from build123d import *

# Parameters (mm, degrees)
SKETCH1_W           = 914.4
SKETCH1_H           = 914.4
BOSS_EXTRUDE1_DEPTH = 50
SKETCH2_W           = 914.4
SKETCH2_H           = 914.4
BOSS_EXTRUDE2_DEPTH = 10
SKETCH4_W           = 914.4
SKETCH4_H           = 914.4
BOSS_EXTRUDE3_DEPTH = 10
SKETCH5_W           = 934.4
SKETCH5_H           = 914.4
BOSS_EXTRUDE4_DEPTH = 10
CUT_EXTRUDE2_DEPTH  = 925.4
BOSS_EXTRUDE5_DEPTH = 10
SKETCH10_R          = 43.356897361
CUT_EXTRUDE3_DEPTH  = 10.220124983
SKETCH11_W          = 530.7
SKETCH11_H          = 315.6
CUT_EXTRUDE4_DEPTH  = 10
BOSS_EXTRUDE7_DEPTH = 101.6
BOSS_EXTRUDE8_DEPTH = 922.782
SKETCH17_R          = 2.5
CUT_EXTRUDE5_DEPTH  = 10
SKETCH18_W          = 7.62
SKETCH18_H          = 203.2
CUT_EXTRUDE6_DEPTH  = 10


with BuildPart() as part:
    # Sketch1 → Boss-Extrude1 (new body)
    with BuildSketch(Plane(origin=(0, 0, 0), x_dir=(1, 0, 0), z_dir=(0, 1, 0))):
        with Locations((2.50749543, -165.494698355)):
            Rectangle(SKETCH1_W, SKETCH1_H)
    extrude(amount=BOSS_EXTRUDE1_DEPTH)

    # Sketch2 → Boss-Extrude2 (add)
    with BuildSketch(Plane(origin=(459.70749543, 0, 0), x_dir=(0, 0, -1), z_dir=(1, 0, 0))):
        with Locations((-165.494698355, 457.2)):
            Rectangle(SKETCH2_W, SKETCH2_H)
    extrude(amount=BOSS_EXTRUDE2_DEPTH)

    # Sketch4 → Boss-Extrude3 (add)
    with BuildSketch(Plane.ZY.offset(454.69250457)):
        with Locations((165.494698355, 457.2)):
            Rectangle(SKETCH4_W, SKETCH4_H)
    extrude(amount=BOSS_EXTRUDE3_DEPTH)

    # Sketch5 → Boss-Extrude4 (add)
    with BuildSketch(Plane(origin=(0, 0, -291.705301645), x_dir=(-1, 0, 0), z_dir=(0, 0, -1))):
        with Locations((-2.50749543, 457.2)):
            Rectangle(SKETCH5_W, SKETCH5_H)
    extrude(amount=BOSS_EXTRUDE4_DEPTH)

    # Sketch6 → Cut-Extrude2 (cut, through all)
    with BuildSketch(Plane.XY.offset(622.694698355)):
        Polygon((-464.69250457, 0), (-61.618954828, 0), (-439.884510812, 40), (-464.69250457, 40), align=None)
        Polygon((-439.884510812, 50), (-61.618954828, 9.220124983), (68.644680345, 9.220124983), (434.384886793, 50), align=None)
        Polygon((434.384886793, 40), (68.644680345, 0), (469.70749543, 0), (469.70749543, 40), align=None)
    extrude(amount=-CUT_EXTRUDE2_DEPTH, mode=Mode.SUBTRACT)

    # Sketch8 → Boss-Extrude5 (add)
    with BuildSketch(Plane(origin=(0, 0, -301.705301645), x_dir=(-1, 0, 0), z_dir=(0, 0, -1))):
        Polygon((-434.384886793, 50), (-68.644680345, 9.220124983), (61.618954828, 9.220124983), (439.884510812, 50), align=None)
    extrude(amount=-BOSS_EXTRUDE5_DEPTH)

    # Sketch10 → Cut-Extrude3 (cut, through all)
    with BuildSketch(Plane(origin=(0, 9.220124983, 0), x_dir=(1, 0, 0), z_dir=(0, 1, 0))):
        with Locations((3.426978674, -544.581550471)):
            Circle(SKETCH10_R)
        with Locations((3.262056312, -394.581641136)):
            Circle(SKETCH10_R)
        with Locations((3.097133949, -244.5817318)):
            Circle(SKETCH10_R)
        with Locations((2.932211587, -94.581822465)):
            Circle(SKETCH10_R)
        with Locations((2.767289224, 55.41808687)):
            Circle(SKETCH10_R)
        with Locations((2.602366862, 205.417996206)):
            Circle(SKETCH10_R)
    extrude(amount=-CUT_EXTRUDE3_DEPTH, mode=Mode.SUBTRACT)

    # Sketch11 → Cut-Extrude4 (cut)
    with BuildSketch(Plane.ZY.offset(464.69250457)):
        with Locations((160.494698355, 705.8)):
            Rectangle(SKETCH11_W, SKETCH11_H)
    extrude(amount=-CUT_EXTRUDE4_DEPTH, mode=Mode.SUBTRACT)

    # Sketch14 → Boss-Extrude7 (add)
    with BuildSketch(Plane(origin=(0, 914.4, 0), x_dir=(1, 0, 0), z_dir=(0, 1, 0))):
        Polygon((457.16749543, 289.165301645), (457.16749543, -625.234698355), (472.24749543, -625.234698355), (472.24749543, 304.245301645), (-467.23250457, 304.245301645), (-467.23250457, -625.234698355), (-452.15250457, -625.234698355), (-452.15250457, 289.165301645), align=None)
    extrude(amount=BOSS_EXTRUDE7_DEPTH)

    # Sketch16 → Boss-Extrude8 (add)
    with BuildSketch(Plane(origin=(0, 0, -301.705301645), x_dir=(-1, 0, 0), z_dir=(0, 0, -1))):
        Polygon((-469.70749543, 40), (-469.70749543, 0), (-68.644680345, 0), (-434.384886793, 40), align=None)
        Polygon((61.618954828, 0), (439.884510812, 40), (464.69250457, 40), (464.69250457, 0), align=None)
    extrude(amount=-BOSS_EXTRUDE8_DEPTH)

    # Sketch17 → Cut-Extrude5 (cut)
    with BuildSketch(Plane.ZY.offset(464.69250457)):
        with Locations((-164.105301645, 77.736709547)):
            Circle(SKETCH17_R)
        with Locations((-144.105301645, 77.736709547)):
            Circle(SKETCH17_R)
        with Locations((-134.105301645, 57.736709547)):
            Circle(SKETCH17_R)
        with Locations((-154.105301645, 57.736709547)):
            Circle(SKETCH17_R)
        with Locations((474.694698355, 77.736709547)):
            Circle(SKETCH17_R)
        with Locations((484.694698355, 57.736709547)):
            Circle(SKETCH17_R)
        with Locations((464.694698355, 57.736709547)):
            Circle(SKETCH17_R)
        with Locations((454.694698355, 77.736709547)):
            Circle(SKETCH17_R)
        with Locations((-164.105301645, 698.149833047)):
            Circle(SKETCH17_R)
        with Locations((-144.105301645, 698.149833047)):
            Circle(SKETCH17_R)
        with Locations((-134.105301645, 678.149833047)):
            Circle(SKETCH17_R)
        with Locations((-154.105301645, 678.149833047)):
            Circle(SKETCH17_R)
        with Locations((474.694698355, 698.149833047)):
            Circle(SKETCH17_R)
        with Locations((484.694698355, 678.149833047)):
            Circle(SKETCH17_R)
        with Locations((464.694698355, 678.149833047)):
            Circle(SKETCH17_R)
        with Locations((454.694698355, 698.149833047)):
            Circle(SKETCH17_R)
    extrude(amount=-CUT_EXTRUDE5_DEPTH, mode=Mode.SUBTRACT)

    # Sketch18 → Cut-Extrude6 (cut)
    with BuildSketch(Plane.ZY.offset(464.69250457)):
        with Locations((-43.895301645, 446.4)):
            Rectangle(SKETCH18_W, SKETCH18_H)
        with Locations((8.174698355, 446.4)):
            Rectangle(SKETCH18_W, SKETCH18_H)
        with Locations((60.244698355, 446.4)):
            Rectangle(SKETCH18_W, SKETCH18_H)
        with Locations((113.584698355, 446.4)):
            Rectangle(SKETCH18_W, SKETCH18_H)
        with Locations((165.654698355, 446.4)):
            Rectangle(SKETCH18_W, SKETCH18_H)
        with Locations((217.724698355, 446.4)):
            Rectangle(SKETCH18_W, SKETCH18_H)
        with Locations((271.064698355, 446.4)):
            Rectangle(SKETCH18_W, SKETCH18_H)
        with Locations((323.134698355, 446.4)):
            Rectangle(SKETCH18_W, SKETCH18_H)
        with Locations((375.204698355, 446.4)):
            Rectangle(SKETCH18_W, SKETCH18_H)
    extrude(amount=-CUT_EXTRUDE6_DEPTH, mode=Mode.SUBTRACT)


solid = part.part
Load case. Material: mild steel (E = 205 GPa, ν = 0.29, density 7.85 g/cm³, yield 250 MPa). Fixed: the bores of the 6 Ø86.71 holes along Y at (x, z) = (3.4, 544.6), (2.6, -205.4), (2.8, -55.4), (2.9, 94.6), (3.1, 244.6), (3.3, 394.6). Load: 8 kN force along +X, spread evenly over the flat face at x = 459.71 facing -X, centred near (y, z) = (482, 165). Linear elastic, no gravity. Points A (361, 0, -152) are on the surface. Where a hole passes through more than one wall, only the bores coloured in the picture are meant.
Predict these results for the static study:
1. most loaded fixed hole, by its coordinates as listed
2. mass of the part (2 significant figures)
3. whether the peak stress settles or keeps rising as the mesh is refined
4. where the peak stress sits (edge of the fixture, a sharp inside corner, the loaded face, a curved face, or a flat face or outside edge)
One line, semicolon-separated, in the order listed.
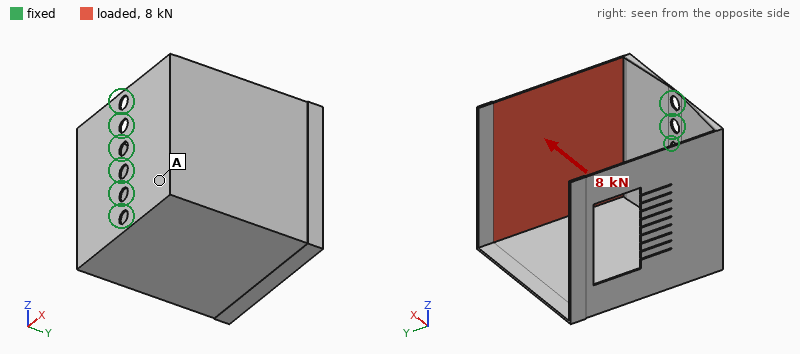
(2.6, -205.4); 400 kg; keeps rising; edge of the fixture
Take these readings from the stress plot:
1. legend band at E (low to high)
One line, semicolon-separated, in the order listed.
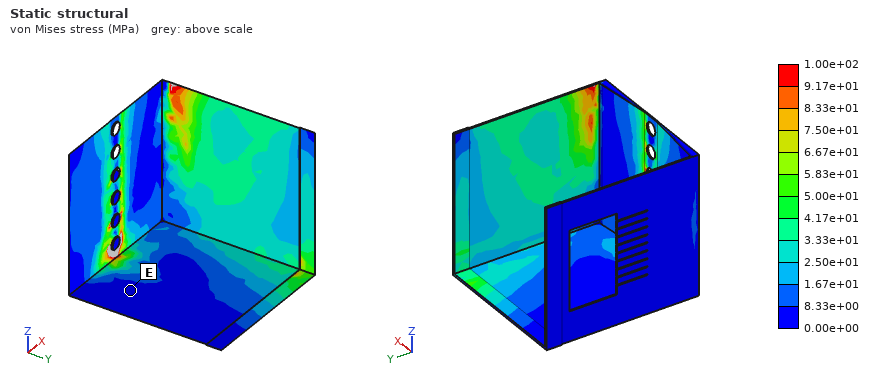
0.00e+00 to 8.33e+00 MPa
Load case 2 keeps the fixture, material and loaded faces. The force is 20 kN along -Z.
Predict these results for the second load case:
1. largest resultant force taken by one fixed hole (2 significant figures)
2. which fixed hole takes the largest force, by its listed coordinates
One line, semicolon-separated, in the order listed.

15 kN; (2.6, -205.4)
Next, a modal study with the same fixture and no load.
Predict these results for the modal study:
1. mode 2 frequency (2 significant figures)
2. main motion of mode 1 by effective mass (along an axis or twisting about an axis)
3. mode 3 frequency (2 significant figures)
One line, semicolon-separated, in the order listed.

16 Hz; along X; 24 Hz
